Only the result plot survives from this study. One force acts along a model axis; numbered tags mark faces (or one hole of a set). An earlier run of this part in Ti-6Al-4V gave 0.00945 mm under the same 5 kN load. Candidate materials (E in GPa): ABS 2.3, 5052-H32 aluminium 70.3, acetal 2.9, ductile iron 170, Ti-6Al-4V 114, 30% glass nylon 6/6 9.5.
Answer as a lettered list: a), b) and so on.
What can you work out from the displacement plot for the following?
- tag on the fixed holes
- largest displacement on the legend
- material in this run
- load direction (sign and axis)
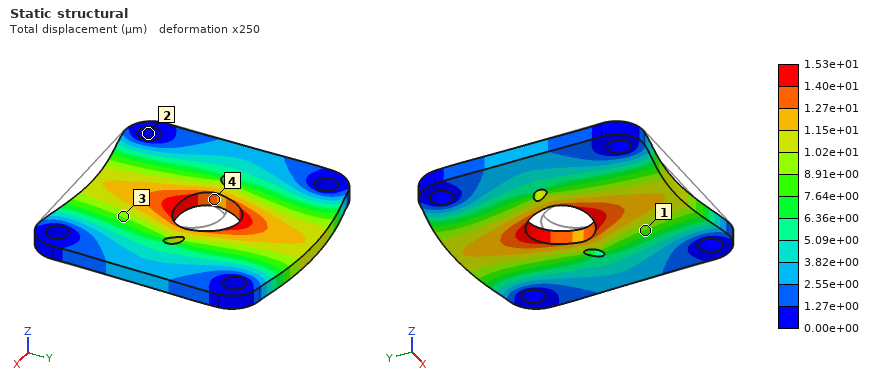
a) 2
b) 1.53e+01 µm
c) 5052-H32 aluminium
d) +Y
